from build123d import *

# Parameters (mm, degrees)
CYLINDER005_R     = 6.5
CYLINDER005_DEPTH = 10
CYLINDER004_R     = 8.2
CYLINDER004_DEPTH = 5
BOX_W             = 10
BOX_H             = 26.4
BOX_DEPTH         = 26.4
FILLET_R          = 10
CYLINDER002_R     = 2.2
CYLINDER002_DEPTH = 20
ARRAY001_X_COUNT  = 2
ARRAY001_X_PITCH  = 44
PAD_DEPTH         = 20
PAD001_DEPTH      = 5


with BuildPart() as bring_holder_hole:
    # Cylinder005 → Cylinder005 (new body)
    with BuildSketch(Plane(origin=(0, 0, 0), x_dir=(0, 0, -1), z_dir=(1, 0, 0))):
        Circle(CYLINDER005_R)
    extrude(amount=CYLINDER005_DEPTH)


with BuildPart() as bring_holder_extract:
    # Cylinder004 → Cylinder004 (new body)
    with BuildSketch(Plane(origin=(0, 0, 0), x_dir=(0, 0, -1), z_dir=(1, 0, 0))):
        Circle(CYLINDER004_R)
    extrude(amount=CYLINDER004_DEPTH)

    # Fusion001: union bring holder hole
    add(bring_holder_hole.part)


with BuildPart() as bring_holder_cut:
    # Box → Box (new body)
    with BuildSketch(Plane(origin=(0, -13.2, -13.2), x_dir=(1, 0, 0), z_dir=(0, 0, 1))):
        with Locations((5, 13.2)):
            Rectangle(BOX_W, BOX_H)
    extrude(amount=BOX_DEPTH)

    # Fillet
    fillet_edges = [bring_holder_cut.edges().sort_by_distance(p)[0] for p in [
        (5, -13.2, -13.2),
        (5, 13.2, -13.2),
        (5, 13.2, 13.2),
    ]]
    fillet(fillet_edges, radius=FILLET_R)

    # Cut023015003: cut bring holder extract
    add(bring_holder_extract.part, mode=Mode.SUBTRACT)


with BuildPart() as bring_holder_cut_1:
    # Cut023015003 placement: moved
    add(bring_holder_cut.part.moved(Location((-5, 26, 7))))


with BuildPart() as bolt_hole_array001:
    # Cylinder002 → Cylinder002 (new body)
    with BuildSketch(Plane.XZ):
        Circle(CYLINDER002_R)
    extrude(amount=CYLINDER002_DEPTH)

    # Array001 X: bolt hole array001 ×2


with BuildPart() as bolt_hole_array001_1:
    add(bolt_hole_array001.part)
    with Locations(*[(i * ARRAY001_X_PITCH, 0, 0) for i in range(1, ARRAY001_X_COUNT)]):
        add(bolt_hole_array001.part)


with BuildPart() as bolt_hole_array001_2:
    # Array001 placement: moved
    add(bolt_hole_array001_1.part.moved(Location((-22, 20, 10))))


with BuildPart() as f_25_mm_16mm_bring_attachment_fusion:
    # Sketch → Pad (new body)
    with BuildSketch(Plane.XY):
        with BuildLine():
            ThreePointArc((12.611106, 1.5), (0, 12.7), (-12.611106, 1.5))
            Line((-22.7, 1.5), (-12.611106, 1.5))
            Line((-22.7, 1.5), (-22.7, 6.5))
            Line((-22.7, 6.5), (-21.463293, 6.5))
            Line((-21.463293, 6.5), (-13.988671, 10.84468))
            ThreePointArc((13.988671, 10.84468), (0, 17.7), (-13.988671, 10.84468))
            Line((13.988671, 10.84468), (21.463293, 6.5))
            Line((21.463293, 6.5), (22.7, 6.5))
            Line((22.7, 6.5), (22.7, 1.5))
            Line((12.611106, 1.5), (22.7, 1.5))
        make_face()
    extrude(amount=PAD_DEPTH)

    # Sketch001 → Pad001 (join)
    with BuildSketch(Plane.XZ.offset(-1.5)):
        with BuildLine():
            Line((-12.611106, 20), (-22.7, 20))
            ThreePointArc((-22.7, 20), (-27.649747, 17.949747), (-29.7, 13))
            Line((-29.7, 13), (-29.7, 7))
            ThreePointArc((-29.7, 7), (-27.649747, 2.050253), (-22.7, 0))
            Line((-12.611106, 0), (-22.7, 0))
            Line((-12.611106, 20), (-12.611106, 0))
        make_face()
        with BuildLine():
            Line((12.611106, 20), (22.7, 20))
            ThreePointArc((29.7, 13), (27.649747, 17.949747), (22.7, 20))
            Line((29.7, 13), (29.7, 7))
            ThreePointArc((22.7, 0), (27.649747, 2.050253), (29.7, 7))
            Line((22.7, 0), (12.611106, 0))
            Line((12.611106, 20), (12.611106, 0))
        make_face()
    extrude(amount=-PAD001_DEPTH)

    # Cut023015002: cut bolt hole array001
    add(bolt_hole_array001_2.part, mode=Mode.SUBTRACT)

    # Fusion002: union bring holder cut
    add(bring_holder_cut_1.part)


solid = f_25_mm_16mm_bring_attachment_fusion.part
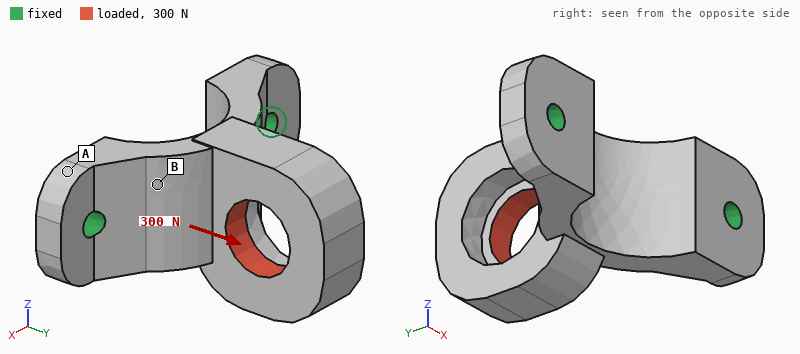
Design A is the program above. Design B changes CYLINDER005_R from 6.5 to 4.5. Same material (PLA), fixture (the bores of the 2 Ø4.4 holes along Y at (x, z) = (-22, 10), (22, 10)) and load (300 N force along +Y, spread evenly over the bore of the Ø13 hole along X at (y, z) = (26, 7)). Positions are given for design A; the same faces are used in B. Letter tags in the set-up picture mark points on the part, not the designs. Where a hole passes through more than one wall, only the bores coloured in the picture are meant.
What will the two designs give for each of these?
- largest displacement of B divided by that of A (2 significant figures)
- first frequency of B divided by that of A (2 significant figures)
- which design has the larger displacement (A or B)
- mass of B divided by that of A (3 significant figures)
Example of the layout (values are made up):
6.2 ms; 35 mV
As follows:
0.91; 0.98; A; 1.03
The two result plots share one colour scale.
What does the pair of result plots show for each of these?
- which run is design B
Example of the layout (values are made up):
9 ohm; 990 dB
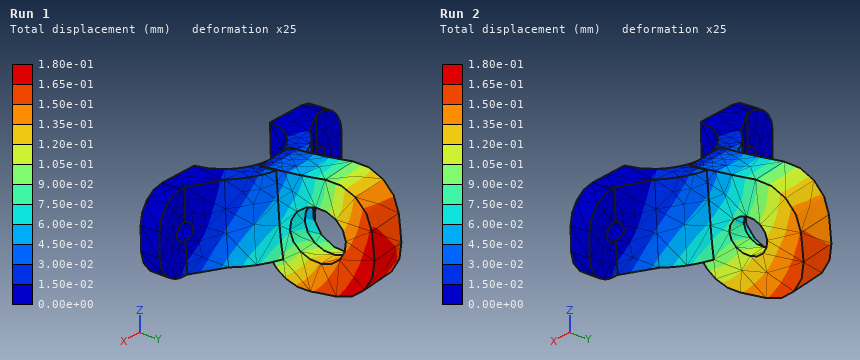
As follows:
Run 2
